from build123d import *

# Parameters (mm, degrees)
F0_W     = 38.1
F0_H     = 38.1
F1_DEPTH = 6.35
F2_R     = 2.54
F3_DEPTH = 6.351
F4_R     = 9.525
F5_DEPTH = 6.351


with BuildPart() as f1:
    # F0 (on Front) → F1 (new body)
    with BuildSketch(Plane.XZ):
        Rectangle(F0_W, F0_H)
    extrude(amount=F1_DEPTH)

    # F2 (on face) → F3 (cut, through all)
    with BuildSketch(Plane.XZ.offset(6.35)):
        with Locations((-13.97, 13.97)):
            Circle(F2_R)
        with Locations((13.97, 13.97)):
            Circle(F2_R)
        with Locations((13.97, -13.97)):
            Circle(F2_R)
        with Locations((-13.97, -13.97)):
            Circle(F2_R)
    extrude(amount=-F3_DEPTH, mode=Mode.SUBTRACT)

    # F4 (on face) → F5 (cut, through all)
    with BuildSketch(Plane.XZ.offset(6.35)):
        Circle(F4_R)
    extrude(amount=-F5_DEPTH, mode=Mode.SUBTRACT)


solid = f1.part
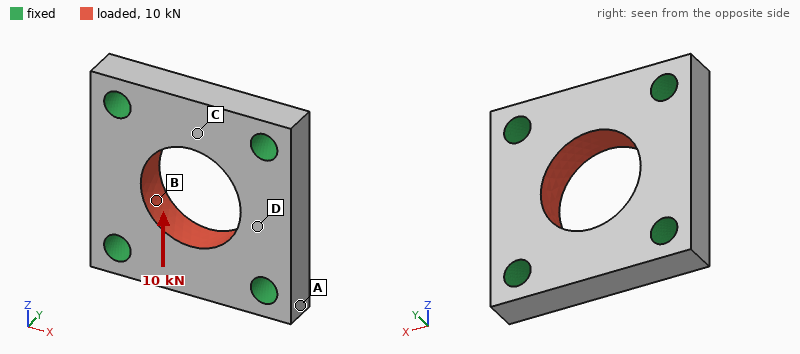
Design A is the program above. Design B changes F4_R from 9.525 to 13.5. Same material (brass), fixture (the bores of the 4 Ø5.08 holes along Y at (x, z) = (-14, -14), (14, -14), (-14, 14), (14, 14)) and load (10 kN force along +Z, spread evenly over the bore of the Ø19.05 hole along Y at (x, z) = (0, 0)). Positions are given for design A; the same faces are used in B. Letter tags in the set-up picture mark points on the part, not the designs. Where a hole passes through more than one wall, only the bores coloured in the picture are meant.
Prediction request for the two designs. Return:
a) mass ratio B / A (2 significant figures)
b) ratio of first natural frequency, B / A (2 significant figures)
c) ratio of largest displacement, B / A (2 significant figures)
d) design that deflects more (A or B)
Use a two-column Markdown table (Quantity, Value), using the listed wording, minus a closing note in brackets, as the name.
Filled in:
| Quantity | Value |
|---|---|
| mass ratio B / A | 0.74 |
| ratio of first natural frequency, B / A | 1.1 |
| ratio of largest displacement, B / A | 1.4 |
| design that deflects more | B |
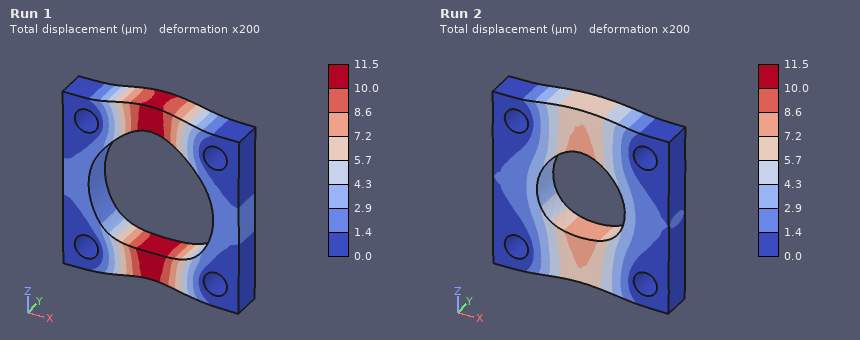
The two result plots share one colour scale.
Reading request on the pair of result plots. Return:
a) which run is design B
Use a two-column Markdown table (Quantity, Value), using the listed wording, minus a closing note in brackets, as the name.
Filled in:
| Quantity | Value |
|---|---|
| which run is design B | Run 1 |
